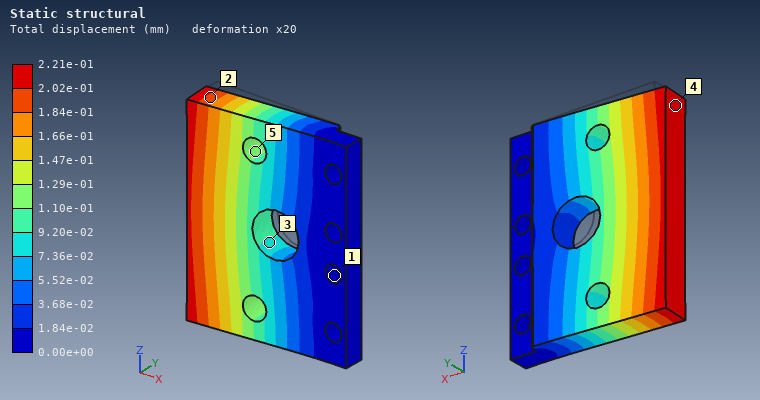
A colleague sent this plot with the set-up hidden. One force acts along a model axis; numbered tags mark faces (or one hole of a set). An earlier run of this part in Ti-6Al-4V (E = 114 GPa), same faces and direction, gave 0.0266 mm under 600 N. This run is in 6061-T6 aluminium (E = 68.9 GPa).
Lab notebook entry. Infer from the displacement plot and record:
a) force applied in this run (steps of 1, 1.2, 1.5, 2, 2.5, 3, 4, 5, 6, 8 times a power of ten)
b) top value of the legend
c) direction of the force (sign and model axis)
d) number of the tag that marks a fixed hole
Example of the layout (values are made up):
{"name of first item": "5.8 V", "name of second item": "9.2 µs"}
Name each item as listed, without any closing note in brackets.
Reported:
{"force applied in this run": "3 kN", "top value of the legend": "2.21e-01 mm", "direction of the force": "-Y", "number of the tag that marks a fixed hole": "1"}
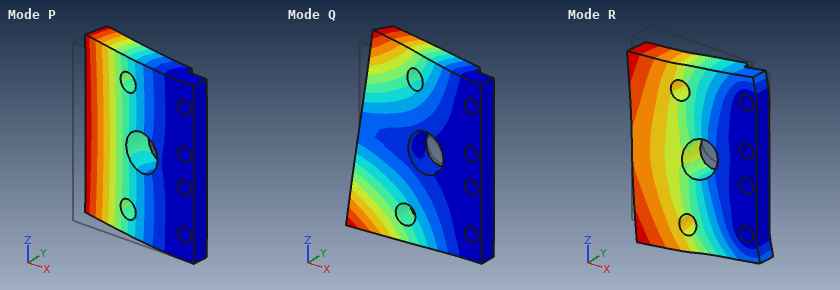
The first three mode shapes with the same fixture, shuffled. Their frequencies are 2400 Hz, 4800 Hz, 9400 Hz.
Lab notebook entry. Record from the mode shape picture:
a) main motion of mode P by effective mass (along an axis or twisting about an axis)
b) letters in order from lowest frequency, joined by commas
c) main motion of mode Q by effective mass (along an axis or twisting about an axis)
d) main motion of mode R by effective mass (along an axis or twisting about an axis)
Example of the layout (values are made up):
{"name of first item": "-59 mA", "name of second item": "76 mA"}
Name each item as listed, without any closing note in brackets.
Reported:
{"main motion of mode P by effective mass": "along Y", "letters in order from lowest frequency, joined by commas": "P, Q, R", "main motion of mode Q by effective mass": "twisting about X", "main motion of mode R by effective mass": "along Z"}
